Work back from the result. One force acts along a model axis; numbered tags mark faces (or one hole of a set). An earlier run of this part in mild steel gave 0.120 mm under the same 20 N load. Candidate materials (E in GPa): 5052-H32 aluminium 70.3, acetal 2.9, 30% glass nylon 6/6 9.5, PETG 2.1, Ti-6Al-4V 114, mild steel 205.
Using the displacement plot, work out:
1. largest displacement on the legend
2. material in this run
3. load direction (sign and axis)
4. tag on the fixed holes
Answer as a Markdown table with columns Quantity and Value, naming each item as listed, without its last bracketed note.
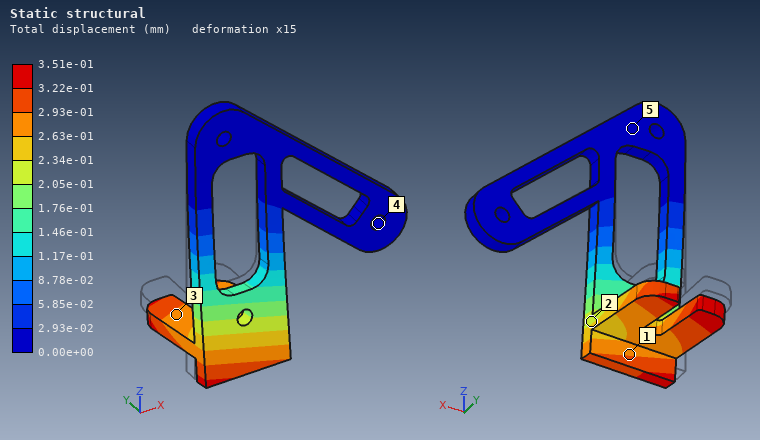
| Quantity | Value |
|---|---|
| largest displacement on the legend | 3.51e-01 mm |
| material in this run | 5052-H32 aluminium |
| load direction | -Y |
| tag on the fixed holes | 4 |
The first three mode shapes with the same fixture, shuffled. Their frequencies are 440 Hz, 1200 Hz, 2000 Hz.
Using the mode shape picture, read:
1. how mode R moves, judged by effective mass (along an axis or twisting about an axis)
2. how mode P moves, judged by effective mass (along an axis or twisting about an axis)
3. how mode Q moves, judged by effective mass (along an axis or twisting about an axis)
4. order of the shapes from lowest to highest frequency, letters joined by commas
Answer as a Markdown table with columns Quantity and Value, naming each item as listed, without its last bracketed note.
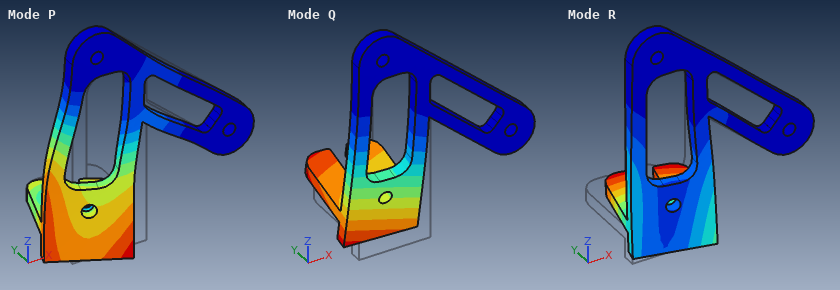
| Quantity | Value |
|---|---|
| how mode R moves, judged by effective mass | along X |
| how mode P moves, judged by effective mass | along X |
| how mode Q moves, judged by effective mass | along Y |
| order of the shapes from lowest to highest frequency, letters joined by commas | Q, R, P |
